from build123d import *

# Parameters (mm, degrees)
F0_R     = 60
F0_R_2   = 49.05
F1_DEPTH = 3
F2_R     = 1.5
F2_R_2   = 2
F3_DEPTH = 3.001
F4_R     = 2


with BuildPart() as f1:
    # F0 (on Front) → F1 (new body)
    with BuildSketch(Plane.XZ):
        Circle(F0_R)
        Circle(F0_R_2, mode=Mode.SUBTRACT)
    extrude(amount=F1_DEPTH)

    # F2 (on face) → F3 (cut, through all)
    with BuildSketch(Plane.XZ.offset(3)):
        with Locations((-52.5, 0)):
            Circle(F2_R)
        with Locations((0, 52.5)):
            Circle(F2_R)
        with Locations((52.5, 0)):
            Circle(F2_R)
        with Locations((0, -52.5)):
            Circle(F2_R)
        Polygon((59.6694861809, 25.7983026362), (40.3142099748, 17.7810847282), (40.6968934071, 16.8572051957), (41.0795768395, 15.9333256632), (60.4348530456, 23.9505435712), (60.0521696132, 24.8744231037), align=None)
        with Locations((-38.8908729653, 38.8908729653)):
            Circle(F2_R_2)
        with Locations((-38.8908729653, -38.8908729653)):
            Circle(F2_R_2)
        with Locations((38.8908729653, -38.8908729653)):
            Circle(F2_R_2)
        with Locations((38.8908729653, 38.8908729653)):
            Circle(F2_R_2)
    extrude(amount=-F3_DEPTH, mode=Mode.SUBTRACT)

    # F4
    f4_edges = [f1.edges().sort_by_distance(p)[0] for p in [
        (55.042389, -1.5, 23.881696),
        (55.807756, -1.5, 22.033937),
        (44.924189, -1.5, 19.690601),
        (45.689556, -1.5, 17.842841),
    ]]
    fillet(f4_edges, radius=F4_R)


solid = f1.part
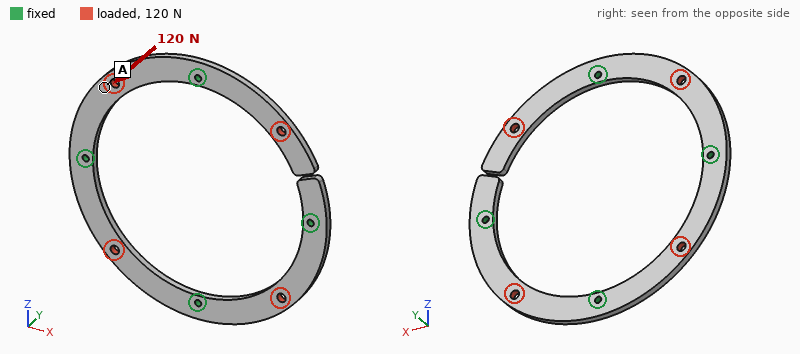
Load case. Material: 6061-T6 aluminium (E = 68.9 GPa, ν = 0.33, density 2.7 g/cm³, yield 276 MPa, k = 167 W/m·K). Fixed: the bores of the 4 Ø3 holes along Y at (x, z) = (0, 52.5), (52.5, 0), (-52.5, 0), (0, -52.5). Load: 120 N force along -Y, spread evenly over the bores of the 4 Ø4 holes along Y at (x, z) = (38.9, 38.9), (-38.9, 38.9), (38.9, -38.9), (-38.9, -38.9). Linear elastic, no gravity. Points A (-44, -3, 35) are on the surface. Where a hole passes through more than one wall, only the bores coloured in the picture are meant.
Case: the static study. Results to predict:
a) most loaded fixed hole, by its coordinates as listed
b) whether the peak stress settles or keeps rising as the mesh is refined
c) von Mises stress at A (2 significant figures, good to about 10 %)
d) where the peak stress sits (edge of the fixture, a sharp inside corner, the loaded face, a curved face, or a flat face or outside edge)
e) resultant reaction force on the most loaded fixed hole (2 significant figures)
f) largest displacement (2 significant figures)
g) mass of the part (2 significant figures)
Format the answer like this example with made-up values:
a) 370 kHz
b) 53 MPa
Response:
a) (0, 52.5)
b) keeps rising
c) 12 MPa
d) edge of the fixture
e) 45 N
f) 0.73 mm
g) 30 g
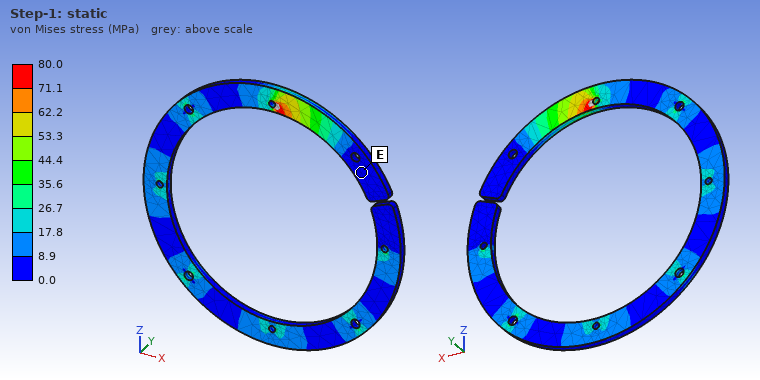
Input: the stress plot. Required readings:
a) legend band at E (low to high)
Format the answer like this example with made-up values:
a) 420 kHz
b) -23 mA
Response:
a) 0.0 to 8.9 MPa
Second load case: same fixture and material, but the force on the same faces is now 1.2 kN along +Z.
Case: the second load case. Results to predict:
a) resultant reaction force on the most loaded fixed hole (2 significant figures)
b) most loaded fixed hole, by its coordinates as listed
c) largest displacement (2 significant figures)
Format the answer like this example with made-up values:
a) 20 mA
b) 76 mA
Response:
a) 490 N
b) (0, 52.5)
c) 0.69 mm
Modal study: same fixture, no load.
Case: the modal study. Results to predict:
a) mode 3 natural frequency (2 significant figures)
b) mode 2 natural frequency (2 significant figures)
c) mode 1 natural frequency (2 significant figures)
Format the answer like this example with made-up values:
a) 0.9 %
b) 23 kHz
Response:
a) 2000 Hz
b) 2000 Hz
c) 660 Hz
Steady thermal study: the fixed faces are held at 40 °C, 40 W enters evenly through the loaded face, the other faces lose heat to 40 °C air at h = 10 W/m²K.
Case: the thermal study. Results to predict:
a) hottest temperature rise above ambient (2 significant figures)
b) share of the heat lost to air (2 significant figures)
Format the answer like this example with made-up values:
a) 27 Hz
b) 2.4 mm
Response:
a) 77 K
b) 5.6 %
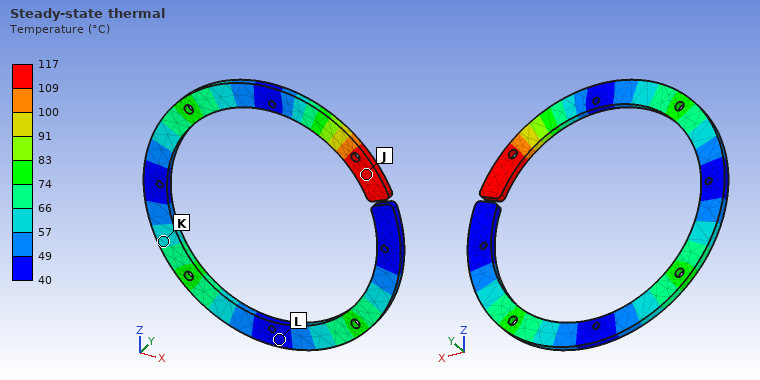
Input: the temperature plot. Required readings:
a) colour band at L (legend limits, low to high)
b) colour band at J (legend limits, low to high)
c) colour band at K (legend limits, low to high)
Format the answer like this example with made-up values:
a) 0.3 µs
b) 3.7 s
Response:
a) 40 to 49 °C
b) 109 to 117 °C
c) 57 to 66 °C
